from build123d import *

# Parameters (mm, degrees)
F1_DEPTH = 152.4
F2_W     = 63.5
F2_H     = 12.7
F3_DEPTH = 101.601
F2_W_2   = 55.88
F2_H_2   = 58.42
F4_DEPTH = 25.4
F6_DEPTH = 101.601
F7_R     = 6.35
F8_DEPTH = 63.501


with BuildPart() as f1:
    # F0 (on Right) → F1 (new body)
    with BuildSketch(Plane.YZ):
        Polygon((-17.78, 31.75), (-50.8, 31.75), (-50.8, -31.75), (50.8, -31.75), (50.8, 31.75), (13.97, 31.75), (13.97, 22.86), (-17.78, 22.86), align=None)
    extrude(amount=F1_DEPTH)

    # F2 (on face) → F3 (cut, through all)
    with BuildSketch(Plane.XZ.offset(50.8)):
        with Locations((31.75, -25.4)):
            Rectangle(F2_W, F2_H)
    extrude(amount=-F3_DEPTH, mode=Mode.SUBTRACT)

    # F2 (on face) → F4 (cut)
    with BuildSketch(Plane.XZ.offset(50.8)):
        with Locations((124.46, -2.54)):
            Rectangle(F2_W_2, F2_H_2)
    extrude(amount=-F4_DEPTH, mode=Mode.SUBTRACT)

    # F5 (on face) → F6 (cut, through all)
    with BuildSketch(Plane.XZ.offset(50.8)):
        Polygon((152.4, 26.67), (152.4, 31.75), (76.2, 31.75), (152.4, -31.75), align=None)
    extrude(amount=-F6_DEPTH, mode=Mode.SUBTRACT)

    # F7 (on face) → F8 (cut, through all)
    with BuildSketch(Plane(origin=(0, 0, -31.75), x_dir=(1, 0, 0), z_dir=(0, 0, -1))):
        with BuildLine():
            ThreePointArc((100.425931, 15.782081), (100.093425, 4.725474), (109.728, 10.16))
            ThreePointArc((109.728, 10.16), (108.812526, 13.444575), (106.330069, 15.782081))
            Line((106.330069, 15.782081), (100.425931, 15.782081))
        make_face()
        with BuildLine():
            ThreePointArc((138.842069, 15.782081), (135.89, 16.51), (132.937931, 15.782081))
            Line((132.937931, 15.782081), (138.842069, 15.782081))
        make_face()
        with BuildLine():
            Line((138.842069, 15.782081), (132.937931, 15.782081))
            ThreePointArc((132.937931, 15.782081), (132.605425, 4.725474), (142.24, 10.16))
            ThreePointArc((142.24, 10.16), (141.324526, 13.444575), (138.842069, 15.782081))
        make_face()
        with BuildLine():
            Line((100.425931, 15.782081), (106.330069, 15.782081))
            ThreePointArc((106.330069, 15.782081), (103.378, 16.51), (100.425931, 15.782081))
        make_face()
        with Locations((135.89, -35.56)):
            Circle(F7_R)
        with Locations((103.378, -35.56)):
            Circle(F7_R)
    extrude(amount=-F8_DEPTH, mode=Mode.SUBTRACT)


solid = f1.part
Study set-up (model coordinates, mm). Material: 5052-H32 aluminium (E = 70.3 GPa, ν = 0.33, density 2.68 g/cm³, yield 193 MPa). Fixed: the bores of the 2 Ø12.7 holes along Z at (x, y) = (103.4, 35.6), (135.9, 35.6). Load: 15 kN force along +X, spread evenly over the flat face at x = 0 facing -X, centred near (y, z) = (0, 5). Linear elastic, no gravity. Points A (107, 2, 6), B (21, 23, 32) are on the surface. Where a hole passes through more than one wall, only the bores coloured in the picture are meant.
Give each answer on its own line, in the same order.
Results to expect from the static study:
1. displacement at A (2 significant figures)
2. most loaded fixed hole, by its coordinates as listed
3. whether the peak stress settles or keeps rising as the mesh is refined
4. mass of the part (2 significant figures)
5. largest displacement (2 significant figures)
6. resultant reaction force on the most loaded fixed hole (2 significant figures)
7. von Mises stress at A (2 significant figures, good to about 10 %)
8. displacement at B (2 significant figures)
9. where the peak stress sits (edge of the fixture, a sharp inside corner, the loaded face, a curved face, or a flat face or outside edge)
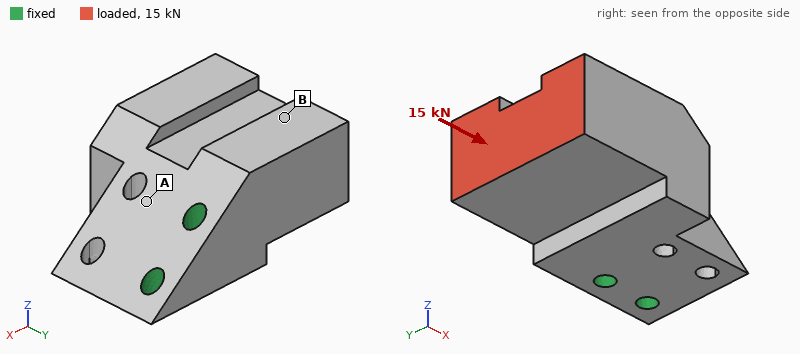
0.024 mm
(103.4, 35.6)
keeps rising
1.6 kg
0.10 mm
15 kN
14 MPa
0.053 mm
edge of the fixture
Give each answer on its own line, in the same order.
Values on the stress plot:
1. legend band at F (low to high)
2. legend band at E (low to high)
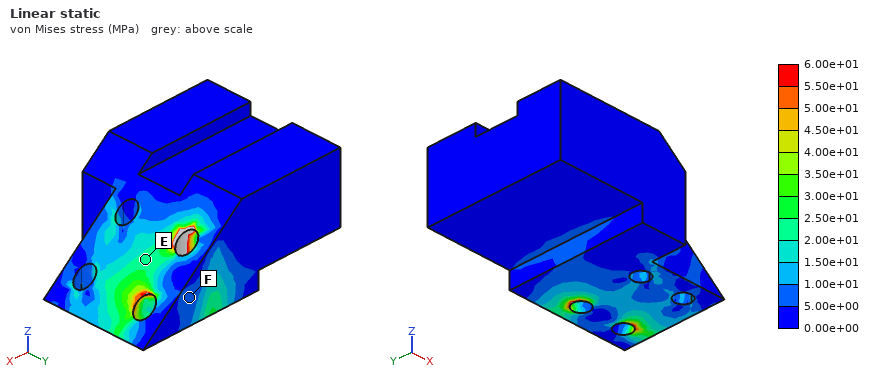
5.00e+00 to 1.00e+01 MPa
2.00e+01 to 2.50e+01 MPa
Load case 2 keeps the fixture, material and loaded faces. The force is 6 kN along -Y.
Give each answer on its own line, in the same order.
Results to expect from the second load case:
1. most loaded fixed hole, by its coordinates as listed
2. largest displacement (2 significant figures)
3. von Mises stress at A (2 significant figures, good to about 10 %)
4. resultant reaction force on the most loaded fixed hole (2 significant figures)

(103.4, 35.6)
0.11 mm
11 MPa
17 kN
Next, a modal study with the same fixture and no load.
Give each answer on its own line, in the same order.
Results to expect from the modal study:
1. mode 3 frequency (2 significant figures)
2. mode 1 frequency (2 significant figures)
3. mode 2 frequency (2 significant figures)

3200 Hz
1600 Hz
1900 Hz
